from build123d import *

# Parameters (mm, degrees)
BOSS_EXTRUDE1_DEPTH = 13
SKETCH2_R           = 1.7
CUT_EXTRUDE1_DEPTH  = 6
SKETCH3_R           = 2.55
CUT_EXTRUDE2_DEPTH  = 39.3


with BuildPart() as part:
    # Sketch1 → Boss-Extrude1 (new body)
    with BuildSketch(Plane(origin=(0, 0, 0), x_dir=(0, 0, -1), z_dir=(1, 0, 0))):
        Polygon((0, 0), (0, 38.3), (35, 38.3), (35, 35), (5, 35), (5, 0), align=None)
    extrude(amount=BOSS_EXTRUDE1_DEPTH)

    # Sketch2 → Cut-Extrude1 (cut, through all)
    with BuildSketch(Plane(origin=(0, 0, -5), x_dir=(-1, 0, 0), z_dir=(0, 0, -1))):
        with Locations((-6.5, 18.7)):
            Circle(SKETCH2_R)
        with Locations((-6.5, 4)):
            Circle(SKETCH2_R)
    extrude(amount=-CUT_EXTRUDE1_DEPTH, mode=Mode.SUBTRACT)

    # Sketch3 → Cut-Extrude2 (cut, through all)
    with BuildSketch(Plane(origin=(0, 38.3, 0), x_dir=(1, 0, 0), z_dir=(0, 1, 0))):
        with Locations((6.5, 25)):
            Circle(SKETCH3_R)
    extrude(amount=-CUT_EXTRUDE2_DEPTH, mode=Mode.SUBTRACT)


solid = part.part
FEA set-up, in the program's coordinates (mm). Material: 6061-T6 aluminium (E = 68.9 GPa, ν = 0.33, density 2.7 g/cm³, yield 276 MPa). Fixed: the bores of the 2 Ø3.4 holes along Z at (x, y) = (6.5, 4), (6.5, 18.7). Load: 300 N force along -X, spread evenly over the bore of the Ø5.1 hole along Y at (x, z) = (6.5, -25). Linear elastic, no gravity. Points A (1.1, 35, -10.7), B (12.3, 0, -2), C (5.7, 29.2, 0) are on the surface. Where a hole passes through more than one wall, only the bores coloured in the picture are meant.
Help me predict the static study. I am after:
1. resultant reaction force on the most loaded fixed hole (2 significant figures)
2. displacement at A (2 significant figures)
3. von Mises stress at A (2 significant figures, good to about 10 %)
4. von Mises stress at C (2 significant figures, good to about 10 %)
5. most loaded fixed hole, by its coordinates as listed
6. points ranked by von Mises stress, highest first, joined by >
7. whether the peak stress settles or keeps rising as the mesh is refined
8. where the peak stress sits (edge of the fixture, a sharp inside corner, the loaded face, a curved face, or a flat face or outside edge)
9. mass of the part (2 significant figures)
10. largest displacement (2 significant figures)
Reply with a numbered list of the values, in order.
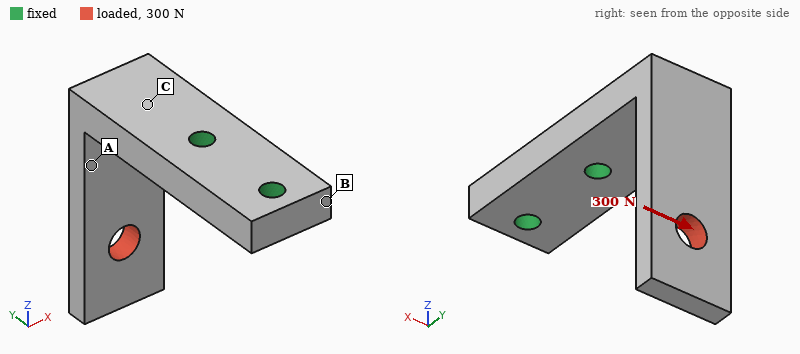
1. 510 N
2. 0.12 mm
3. 49 MPa
4. 110 MPa
5. (6.5, 18.7)
6. C > A > B
7. keeps rising
8. edge of the fixture
9. 9.8 g
10. 0.41 mm
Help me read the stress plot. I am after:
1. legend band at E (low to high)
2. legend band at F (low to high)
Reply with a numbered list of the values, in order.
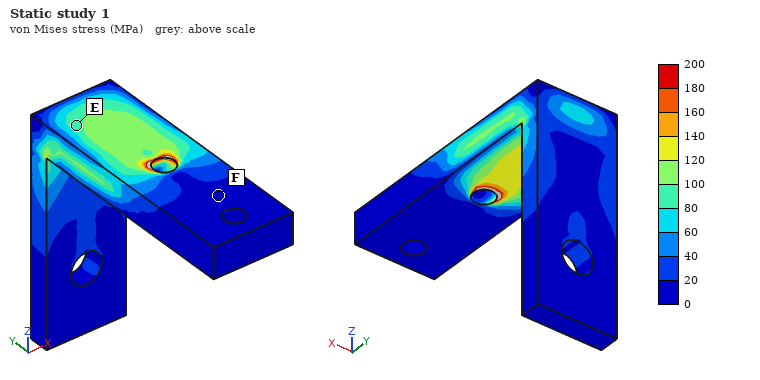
1. 80 to 100 MPa
2. 0 to 20 MPa
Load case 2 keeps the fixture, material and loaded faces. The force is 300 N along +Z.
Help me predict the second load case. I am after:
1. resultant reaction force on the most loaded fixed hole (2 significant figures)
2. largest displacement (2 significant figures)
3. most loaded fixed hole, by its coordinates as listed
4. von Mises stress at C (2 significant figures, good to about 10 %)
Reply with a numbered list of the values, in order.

1. 370 N
2. 0.18 mm
3. (6.5, 18.7)
4. 39 MPa
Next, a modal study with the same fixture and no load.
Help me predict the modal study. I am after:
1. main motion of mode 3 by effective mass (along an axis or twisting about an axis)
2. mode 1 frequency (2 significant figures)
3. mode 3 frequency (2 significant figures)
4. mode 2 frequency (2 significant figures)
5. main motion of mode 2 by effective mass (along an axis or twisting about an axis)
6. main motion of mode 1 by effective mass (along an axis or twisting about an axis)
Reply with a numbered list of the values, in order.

1. along Z
2. 2100 Hz
3. 6200 Hz
4. 3300 Hz
5. along X
6. along Y
